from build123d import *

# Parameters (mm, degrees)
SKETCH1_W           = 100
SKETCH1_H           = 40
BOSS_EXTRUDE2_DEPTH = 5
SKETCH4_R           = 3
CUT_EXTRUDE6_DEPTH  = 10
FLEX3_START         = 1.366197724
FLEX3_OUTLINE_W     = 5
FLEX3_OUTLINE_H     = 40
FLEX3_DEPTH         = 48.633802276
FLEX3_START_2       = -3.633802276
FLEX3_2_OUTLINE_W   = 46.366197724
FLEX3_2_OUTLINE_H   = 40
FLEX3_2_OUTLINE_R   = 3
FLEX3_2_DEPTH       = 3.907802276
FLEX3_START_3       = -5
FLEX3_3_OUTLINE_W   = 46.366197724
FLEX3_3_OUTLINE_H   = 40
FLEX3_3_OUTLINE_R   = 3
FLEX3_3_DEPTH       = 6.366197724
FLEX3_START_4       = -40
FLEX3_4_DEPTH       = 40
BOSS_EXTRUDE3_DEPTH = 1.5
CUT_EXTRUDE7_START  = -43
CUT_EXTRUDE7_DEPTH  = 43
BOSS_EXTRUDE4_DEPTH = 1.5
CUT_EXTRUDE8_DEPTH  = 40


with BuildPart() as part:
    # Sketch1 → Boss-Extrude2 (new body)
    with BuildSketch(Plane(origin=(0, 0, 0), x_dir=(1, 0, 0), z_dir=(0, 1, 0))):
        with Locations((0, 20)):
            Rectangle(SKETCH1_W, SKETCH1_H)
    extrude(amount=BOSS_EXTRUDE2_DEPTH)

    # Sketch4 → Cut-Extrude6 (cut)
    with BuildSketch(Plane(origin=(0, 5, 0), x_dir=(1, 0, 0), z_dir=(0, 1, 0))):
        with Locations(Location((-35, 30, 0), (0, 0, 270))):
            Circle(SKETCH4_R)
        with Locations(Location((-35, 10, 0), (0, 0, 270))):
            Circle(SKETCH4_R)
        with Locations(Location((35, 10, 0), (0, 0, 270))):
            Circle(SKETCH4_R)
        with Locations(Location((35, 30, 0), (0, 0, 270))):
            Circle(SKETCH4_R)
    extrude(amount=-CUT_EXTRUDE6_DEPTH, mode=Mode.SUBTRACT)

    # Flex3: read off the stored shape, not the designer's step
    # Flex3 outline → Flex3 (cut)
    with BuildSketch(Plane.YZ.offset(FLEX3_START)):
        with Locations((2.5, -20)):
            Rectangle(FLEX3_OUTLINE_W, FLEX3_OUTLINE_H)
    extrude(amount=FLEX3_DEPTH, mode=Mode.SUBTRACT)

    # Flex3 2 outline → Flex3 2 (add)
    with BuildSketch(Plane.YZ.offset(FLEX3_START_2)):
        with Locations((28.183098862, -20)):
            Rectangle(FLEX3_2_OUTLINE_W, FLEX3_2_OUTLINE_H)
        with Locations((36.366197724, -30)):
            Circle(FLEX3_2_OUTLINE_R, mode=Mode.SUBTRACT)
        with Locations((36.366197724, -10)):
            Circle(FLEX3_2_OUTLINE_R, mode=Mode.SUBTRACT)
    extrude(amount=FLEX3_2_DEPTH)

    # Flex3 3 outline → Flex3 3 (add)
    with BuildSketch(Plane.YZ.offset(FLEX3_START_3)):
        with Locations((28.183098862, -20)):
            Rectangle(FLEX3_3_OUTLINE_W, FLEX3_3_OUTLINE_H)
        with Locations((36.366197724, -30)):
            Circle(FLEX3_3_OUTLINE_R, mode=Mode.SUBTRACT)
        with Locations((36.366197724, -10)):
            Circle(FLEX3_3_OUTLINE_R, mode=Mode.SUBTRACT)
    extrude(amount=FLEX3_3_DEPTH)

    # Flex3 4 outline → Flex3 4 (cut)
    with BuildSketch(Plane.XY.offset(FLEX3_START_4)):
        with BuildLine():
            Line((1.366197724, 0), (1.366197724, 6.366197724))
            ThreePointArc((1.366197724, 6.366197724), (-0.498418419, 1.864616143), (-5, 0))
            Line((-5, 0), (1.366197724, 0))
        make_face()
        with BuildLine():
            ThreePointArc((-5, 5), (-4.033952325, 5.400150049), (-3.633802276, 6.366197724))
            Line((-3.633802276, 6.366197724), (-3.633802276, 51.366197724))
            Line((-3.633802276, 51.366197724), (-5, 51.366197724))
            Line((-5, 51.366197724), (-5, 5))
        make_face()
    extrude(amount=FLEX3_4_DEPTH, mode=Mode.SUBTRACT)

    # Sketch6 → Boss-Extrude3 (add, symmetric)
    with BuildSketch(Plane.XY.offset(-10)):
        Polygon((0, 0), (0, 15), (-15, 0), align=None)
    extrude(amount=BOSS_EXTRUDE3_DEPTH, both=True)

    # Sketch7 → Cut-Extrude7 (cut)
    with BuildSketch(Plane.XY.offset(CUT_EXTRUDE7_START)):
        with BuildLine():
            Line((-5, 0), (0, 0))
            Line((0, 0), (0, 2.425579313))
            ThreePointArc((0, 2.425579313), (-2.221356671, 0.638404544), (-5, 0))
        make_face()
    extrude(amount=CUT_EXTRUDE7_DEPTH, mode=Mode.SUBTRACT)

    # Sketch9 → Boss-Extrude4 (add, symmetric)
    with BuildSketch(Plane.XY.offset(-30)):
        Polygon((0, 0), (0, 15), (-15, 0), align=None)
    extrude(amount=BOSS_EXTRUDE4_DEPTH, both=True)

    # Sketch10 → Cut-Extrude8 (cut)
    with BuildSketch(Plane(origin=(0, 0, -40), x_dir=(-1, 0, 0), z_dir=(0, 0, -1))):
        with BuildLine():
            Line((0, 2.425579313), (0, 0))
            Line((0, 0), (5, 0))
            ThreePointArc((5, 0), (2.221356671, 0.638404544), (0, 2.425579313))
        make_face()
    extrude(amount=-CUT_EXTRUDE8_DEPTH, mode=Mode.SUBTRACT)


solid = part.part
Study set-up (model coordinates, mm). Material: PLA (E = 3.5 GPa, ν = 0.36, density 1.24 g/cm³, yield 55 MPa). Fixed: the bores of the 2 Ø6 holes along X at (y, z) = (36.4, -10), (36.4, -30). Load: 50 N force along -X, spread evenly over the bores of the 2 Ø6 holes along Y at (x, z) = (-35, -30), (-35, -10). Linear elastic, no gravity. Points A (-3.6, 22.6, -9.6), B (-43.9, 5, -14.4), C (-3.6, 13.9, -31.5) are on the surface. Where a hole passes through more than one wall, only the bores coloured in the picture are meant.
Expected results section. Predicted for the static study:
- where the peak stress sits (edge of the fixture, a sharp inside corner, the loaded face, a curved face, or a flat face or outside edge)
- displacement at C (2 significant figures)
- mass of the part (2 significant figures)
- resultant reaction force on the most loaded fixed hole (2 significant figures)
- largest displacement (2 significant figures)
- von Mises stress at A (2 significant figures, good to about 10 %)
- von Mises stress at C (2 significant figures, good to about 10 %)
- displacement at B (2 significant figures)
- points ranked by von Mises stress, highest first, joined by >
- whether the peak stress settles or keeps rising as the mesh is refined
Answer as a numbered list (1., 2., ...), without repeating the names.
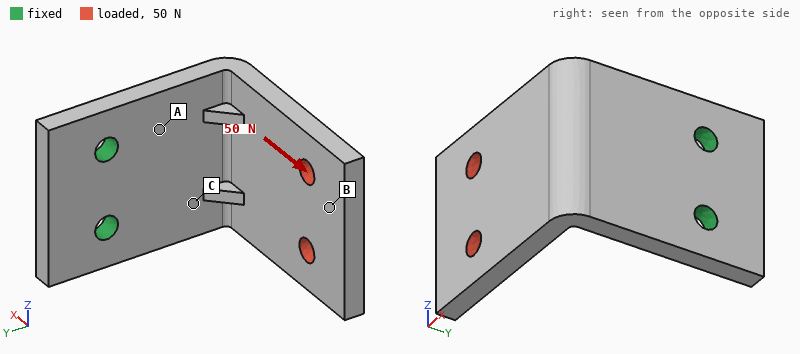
1. edge of the fixture
2. 0.19 mm
3. 23 g
4. 25 N
5. 0.93 mm
6. 5.4 MPa
7. 3.3 MPa
8. 0.80 mm
9. A > C > B
10. keeps rising
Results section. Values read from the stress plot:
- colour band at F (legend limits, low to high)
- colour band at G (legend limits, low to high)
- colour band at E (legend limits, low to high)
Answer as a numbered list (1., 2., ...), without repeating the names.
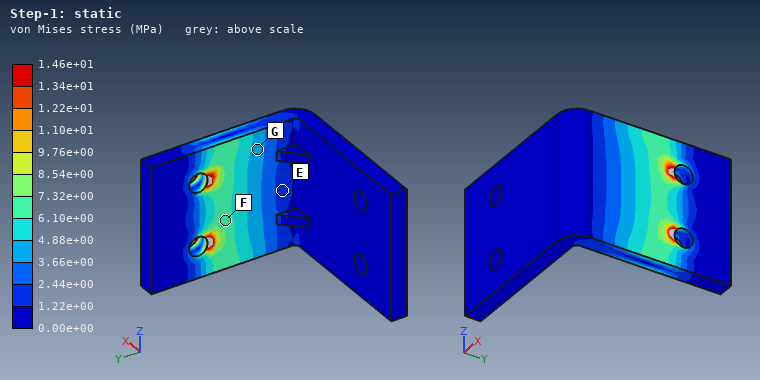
1. 6.10e+00 to 7.32e+00 MPa
2. 3.66e+00 to 4.88e+00 MPa
3. 1.22e+00 to 2.44e+00 MPa
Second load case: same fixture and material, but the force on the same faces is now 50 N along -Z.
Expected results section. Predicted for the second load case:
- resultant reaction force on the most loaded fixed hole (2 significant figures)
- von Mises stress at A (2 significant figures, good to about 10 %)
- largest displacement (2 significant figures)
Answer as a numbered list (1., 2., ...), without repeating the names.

1. 97 N
2. 6.3 MPa
3. 0.86 mm
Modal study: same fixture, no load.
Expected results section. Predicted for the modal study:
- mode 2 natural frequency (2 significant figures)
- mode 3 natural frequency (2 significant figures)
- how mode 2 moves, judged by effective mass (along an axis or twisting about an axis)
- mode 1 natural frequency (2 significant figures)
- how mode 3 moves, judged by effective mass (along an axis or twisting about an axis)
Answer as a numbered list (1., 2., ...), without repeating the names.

1. 490 Hz
2. 890 Hz
3. along Z
4. 290 Hz
5. along X
